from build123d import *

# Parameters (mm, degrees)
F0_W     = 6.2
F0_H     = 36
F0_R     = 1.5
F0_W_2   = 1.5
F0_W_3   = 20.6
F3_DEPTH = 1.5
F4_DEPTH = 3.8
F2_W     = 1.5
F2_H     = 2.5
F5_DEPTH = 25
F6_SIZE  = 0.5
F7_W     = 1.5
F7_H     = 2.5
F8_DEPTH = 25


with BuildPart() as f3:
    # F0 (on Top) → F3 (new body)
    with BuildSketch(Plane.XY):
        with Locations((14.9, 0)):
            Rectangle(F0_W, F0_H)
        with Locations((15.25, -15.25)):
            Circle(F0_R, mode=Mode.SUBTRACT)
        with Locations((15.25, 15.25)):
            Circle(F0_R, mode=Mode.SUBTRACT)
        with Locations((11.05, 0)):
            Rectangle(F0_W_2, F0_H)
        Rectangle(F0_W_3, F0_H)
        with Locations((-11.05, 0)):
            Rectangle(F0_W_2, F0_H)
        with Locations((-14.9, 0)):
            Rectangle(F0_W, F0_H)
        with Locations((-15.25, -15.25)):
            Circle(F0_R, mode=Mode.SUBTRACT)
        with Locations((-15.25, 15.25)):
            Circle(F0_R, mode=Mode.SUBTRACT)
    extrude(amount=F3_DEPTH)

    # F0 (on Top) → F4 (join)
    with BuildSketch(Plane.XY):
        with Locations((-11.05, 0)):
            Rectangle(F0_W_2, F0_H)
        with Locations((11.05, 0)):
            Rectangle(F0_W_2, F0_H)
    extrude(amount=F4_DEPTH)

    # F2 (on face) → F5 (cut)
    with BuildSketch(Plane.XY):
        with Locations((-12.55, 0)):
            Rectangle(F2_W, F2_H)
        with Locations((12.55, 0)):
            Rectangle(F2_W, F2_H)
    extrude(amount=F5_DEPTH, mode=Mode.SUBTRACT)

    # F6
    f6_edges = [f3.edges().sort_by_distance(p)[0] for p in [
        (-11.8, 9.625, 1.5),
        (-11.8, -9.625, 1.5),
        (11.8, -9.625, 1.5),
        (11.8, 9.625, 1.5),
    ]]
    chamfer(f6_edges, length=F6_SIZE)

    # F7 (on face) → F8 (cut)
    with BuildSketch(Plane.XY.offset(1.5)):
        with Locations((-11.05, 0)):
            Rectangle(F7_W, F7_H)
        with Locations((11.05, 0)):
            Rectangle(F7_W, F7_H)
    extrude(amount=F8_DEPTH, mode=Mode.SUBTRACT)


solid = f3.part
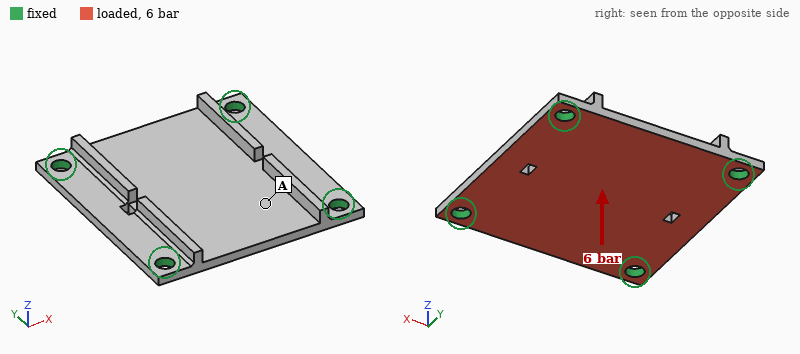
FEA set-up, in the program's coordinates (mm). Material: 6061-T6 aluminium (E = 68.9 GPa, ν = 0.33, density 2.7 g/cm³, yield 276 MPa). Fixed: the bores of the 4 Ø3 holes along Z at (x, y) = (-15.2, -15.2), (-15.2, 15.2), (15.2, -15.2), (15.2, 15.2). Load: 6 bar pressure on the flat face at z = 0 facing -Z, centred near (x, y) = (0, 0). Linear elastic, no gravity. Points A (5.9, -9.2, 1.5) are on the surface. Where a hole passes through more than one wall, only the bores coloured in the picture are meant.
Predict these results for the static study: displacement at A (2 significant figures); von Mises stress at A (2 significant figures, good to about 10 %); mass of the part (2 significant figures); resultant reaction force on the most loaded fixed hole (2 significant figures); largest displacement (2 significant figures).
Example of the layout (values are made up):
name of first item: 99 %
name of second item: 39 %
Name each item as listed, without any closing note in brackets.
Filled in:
displacement at A: 0.086 mm
von Mises stress at A: 40 MPa
mass of the part: 5.8 g
resultant reaction force on the most loaded fixed hole: 190 N
largest displacement: 0.13 mm
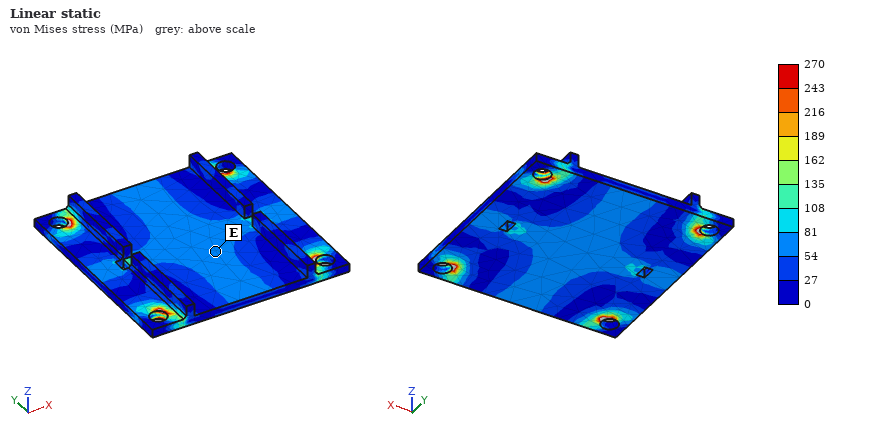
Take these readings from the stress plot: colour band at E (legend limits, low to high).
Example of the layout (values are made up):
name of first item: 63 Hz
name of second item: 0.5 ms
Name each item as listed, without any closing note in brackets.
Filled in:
colour band at E: 54 to 81 MPa
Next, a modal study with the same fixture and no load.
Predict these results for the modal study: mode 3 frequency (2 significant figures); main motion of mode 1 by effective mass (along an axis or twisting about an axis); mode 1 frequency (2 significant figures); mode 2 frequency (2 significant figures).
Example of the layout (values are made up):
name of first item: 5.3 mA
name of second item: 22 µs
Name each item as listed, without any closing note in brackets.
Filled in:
mode 3 frequency: 11 kHz
main motion of mode 1 by effective mass: along Z
mode 1 frequency: 6300 Hz
mode 2 frequency: 11 kHz
